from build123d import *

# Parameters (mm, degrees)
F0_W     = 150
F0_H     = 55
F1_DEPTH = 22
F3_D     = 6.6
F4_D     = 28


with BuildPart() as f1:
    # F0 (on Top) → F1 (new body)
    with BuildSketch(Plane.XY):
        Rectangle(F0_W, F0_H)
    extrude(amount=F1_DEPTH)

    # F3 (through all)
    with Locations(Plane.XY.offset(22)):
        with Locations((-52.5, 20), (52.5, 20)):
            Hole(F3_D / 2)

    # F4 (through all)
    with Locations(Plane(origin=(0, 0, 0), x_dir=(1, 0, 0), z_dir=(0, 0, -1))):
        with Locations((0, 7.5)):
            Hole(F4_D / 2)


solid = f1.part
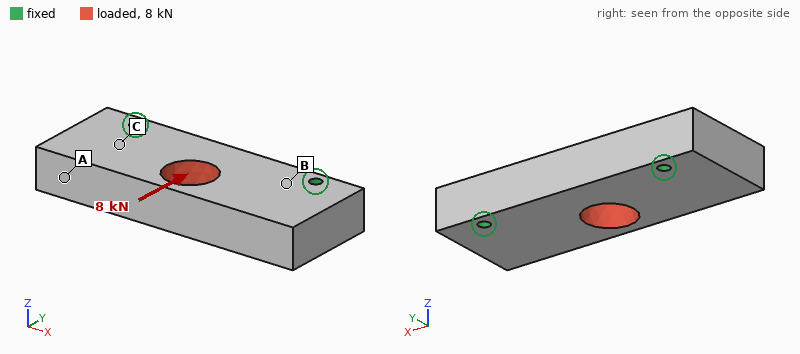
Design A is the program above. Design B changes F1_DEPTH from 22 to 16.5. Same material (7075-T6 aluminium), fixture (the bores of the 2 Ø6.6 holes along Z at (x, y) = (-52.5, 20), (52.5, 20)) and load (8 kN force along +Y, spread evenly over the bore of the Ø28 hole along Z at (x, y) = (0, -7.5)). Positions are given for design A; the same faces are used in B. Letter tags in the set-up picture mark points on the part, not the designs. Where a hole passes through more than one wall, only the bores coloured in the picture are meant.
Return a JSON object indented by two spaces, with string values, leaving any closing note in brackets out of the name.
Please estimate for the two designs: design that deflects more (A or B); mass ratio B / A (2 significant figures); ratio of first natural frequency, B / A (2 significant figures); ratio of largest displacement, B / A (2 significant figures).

{
  "design that deflects more": "B",
  "mass ratio B / A": "0.75",
  "ratio of first natural frequency, B / A": "0.82",
  "ratio of largest displacement, B / A": "1.3"
}
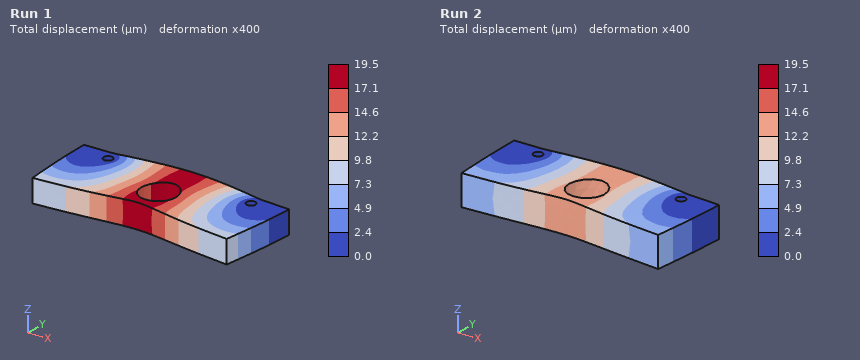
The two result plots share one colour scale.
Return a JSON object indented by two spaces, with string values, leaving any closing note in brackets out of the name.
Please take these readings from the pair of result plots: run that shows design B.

{
  "run that shows design B": "Run 1"
}
